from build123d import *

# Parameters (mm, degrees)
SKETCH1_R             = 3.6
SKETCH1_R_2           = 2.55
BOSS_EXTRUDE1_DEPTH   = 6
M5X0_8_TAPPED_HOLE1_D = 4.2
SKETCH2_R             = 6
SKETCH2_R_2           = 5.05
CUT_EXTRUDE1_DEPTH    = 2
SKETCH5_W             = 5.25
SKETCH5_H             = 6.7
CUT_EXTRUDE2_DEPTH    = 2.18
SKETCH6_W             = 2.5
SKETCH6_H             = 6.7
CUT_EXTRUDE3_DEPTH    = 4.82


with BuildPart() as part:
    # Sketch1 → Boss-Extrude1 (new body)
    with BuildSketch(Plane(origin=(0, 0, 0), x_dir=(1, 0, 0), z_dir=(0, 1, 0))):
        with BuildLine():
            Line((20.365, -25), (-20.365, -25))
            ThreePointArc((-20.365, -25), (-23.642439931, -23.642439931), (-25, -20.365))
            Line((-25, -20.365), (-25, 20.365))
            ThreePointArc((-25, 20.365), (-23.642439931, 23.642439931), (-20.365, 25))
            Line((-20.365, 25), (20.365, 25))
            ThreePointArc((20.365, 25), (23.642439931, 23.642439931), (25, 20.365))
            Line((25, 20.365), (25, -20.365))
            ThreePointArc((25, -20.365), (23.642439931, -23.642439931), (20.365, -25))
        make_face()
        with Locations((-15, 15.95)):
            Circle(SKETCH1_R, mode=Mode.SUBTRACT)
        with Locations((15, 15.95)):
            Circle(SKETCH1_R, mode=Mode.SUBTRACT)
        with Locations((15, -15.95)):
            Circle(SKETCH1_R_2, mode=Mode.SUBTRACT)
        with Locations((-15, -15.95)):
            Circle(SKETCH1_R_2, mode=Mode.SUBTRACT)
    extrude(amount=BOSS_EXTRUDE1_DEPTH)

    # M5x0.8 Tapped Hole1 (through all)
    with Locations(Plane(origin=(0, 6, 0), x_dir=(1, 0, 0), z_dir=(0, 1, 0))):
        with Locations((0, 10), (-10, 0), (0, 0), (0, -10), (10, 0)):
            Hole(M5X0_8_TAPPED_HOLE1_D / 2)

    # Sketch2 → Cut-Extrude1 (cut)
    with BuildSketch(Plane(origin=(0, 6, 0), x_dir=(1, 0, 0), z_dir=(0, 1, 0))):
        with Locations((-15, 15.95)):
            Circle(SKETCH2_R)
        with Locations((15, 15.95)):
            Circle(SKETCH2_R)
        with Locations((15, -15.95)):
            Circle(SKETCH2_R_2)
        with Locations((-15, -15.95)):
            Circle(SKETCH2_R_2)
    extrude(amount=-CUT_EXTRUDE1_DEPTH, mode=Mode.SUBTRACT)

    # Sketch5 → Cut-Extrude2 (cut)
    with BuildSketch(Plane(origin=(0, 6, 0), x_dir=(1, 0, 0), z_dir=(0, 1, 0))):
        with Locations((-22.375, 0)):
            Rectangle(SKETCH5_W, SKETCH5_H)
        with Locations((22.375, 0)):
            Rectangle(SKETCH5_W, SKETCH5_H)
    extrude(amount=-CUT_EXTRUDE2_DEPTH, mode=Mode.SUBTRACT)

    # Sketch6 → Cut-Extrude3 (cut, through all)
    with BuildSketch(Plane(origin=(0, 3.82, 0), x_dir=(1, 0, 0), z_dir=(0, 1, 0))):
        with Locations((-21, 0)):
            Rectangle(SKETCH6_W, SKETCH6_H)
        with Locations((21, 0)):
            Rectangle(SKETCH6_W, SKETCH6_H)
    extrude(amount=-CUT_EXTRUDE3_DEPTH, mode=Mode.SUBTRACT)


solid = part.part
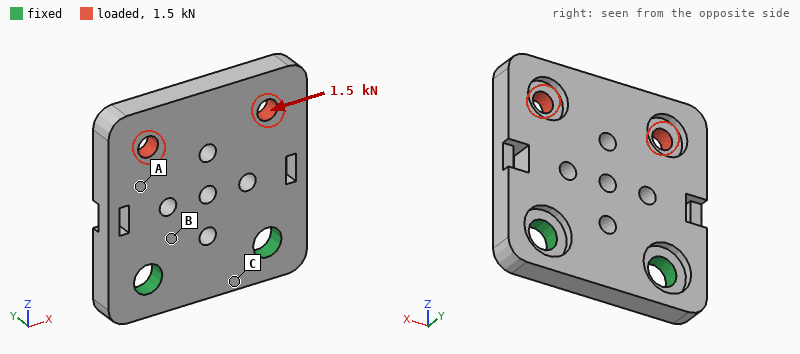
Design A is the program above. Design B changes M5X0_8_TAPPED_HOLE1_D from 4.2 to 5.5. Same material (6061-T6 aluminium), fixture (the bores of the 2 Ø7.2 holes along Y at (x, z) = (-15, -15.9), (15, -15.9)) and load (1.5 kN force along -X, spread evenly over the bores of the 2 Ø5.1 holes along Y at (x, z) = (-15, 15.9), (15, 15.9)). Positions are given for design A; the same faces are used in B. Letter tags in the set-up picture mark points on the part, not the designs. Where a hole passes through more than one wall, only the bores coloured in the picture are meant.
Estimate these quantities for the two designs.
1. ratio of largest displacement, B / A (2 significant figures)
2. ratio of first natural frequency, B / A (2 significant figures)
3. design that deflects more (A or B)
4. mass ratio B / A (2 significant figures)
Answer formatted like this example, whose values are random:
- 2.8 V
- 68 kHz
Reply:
- 1.1
- 0.98
- B
- 0.98
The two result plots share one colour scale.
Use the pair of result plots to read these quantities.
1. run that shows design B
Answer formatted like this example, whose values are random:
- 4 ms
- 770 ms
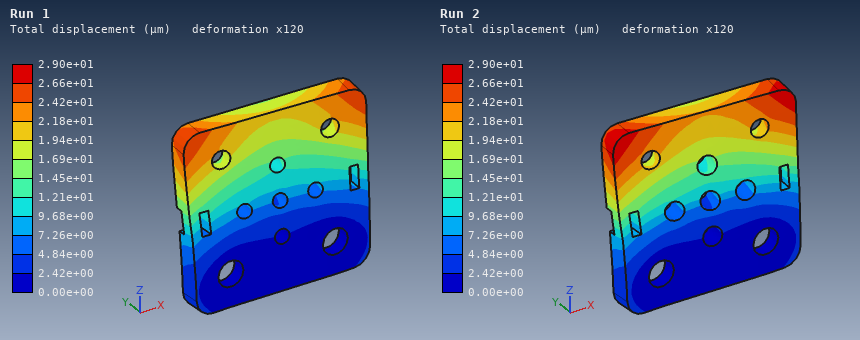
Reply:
- Run 2
